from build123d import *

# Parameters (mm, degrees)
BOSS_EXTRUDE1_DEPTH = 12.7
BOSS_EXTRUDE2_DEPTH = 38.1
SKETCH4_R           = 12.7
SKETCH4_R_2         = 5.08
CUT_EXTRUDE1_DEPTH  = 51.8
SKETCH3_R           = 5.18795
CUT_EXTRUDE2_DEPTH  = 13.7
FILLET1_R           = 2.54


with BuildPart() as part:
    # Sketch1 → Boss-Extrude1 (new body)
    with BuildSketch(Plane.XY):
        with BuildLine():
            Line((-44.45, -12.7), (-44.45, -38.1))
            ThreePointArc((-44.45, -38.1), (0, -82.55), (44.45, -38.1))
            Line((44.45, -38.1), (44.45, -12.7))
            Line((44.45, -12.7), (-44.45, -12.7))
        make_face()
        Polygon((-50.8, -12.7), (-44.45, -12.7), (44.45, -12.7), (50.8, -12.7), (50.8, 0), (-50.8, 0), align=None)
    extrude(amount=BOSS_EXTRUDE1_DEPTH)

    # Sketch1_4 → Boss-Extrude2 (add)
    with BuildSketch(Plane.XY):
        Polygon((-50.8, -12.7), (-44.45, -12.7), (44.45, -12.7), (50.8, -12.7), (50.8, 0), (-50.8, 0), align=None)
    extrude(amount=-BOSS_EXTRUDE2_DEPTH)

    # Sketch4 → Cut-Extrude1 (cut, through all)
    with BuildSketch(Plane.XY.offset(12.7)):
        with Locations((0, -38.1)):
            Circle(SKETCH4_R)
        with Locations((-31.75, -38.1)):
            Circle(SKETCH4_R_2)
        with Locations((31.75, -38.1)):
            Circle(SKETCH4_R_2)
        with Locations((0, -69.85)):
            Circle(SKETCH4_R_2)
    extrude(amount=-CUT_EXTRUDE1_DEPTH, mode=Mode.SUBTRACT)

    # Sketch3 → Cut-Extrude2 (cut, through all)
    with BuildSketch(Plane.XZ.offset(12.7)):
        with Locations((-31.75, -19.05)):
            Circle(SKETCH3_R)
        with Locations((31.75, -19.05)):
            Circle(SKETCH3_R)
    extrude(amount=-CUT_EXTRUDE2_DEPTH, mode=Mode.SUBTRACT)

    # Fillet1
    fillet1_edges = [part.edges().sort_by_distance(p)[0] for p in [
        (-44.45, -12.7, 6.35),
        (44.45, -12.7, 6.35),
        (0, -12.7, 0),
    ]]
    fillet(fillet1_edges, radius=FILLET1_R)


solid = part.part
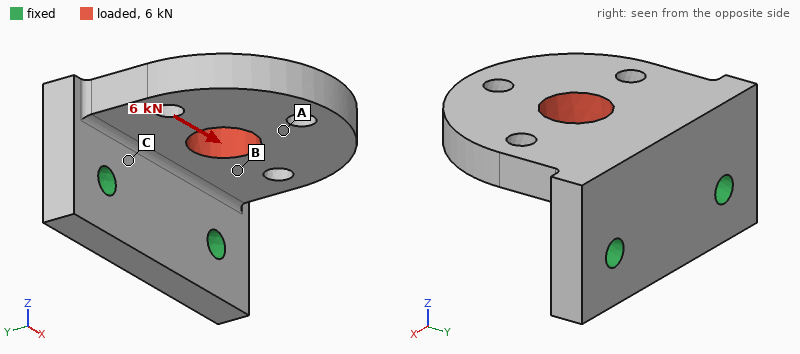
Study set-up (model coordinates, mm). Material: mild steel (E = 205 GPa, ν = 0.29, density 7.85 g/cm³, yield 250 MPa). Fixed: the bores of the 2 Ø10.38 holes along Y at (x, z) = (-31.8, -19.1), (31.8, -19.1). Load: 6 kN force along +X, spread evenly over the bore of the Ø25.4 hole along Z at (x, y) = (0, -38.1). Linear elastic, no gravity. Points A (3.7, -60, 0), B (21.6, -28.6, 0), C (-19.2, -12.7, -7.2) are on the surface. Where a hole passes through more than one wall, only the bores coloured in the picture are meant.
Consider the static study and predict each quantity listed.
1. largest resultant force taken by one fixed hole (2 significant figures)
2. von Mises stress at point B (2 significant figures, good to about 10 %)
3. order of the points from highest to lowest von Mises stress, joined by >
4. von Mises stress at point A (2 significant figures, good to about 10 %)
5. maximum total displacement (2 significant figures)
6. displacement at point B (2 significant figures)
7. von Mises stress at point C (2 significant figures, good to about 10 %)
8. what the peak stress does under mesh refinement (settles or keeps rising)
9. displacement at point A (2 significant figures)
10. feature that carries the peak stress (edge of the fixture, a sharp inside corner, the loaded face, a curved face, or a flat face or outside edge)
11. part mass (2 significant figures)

4.5 kN
16 MPa
C > B > A
6.6 MPa
22 µm
9.2 µm
27 MPa
keeps rising
18 µm
edge of the fixture
960 g
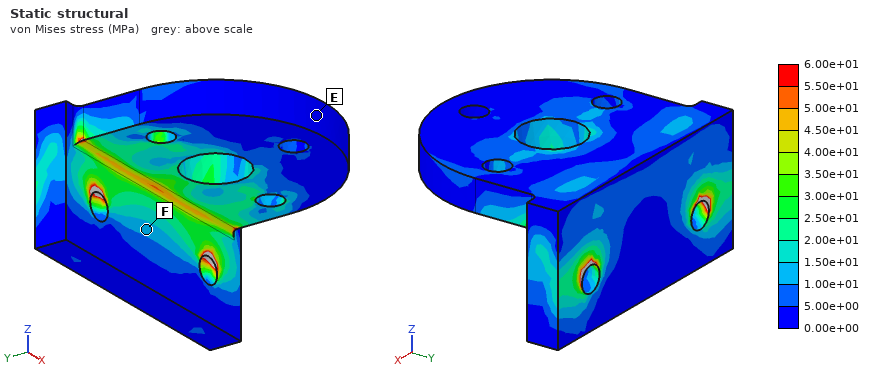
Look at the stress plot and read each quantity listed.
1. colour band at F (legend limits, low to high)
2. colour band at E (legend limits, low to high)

1.00e+01 to 1.50e+01 MPa
0.00e+00 to 5.00e+00 MPa
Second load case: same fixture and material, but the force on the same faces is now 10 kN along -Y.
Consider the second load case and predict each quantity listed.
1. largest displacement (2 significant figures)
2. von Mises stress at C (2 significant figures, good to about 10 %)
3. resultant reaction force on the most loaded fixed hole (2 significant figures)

83 µm
40 MPa
5.0 kN
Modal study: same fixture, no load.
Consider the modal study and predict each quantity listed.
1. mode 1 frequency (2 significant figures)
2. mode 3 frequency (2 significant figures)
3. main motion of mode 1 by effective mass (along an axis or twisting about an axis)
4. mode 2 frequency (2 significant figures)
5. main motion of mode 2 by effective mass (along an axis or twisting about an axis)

1500 Hz
5100 Hz
along Z
3500 Hz
along X
